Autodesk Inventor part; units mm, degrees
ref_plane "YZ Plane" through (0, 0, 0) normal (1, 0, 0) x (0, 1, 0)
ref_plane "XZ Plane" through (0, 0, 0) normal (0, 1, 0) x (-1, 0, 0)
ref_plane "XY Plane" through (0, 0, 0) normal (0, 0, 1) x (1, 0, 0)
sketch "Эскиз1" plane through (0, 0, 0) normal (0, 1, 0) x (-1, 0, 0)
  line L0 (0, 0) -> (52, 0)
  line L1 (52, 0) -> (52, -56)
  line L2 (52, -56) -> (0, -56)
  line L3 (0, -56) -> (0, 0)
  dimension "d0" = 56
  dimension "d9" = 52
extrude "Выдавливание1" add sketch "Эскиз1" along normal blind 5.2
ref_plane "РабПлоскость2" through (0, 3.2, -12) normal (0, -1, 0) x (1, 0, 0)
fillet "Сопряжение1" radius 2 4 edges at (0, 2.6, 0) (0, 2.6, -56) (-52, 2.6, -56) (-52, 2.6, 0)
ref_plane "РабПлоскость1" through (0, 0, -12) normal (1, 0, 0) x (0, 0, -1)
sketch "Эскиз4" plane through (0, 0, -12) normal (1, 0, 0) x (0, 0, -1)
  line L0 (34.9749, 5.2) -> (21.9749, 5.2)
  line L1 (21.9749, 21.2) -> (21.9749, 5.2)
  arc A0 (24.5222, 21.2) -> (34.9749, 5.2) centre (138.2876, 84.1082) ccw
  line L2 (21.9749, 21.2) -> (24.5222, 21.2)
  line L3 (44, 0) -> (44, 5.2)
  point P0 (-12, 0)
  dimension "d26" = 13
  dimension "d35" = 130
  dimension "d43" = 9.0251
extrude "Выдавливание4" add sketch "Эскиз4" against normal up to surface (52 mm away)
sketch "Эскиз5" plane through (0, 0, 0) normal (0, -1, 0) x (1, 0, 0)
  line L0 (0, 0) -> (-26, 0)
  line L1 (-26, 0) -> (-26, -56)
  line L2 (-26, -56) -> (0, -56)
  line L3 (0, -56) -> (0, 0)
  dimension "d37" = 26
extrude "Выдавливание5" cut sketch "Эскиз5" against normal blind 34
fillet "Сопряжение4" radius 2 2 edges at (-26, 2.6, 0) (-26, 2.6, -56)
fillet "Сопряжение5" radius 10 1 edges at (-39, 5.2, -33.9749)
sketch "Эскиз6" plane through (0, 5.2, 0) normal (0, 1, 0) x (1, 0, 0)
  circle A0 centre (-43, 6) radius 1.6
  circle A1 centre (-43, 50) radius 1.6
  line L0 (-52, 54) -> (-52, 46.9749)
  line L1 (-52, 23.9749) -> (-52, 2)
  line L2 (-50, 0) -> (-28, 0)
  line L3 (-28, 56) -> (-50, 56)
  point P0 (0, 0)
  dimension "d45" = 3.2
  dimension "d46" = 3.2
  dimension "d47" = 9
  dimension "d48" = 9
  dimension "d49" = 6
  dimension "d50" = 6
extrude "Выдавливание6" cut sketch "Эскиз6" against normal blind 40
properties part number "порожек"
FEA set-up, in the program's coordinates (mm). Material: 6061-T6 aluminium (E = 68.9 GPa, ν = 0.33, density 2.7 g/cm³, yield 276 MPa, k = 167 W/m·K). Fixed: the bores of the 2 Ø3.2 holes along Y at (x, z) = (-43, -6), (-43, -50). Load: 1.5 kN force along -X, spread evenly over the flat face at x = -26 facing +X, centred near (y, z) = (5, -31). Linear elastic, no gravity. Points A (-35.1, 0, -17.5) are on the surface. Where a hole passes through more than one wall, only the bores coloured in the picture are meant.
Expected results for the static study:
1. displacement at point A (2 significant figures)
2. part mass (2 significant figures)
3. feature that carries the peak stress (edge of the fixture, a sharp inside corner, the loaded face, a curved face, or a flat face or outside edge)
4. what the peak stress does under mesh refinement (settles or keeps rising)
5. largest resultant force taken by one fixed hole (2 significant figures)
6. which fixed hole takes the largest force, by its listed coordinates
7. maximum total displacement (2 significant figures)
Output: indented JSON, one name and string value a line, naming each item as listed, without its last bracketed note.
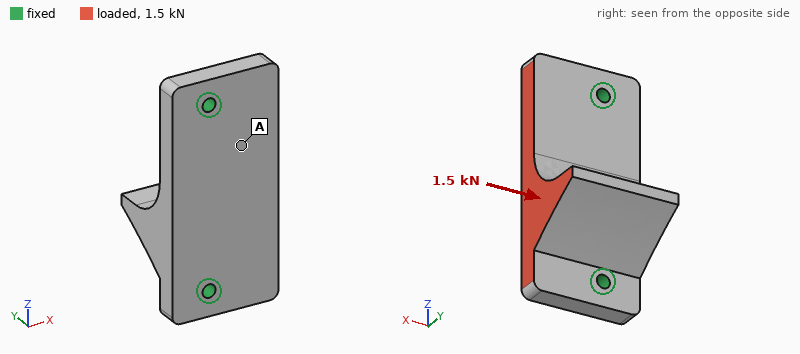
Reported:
{
  "displacement at point A": "4.7 µm",
  "part mass": "30 g",
  "feature that carries the peak stress": "edge of the fixture",
  "what the peak stress does under mesh refinement": "keeps rising",
  "largest resultant force taken by one fixed hole": "890 N",
  "which fixed hole takes the largest force, by its listed coordinates": "(-43, -50)",
  "maximum total displacement": "28 µm"
}
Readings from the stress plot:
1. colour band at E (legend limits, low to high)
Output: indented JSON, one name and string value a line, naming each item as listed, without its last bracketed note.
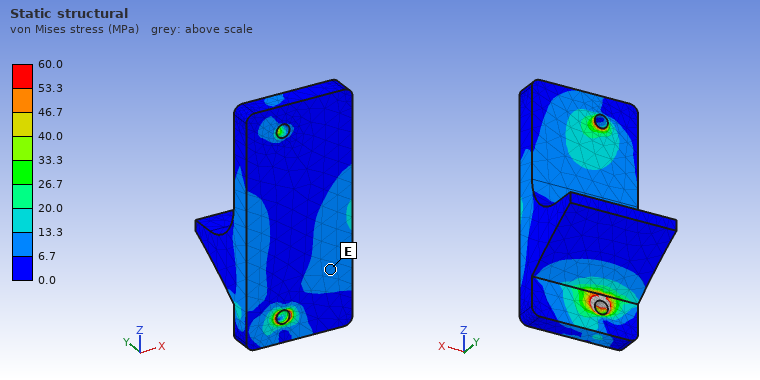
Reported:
{
  "colour band at E": "6.7 to 13.3 MPa"
}
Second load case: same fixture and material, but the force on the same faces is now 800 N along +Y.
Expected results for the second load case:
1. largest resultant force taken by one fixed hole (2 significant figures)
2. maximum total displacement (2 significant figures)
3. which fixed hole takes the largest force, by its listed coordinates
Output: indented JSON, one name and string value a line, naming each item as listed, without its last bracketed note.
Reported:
{
  "largest resultant force taken by one fixed hole": "460 N",
  "maximum total displacement": "73 µm",
  "which fixed hole takes the largest force, by its listed coordinates": "(-43, -50)"
}
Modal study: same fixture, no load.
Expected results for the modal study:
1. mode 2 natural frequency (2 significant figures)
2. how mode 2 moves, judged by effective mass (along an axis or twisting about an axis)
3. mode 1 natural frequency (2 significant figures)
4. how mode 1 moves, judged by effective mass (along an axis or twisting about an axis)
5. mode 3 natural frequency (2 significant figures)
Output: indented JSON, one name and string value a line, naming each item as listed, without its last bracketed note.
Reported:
{
  "mode 2 natural frequency": "9400 Hz",
  "how mode 2 moves, judged by effective mass": "along Y",
  "mode 1 natural frequency": "6400 Hz",
  "how mode 1 moves, judged by effective mass": "along Y",
  "mode 3 natural frequency": "16 kHz"
}
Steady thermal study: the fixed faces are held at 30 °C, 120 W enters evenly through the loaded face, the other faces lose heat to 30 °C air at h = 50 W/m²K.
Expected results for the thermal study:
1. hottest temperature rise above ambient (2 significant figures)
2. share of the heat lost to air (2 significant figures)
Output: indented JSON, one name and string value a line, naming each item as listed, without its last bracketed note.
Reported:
{
  "hottest temperature rise above ambient": "58 K",
  "share of the heat lost to air": "5.0 %"
}
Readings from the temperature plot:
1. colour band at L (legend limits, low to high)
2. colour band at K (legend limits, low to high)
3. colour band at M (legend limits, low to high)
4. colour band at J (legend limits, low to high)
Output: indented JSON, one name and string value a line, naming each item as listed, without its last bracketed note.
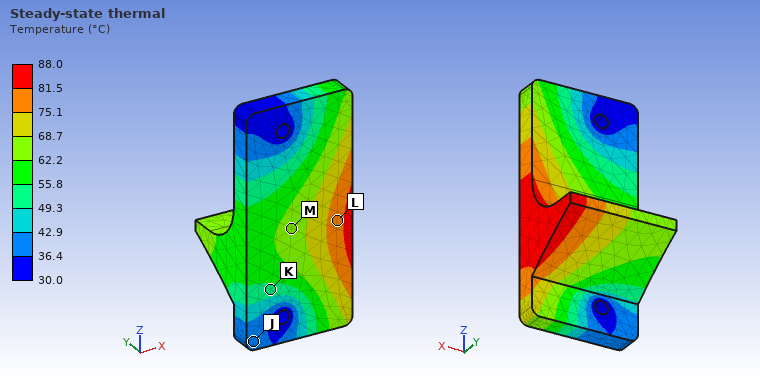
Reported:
{
  "colour band at L": "75.1 to 81.5 °C",
  "colour band at K": "49.3 to 55.8 °C",
  "colour band at M": "62.2 to 68.7 °C",
  "colour band at J": "36.4 to 42.9 °C"
}
